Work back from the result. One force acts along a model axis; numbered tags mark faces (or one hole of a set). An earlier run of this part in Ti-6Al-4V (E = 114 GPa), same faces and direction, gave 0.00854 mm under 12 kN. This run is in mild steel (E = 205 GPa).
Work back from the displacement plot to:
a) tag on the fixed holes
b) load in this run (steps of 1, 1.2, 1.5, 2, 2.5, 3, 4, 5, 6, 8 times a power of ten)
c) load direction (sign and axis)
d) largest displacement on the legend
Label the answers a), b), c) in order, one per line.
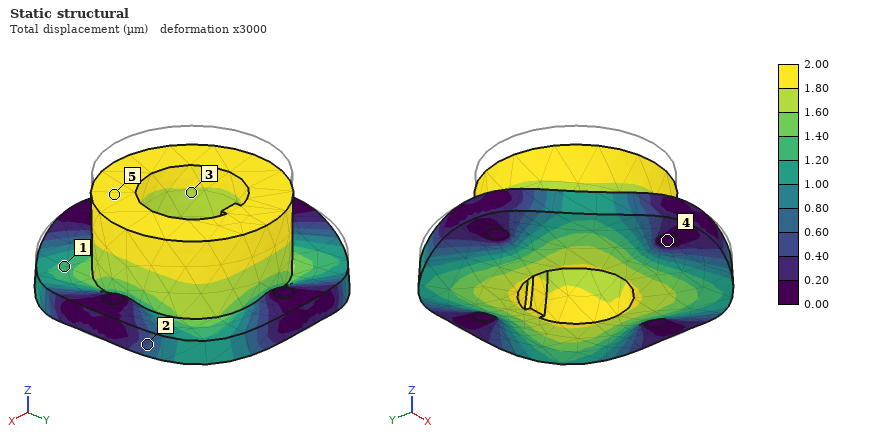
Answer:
a) 4
b) 5 kN
c) -Z
d) 2.00 µm
